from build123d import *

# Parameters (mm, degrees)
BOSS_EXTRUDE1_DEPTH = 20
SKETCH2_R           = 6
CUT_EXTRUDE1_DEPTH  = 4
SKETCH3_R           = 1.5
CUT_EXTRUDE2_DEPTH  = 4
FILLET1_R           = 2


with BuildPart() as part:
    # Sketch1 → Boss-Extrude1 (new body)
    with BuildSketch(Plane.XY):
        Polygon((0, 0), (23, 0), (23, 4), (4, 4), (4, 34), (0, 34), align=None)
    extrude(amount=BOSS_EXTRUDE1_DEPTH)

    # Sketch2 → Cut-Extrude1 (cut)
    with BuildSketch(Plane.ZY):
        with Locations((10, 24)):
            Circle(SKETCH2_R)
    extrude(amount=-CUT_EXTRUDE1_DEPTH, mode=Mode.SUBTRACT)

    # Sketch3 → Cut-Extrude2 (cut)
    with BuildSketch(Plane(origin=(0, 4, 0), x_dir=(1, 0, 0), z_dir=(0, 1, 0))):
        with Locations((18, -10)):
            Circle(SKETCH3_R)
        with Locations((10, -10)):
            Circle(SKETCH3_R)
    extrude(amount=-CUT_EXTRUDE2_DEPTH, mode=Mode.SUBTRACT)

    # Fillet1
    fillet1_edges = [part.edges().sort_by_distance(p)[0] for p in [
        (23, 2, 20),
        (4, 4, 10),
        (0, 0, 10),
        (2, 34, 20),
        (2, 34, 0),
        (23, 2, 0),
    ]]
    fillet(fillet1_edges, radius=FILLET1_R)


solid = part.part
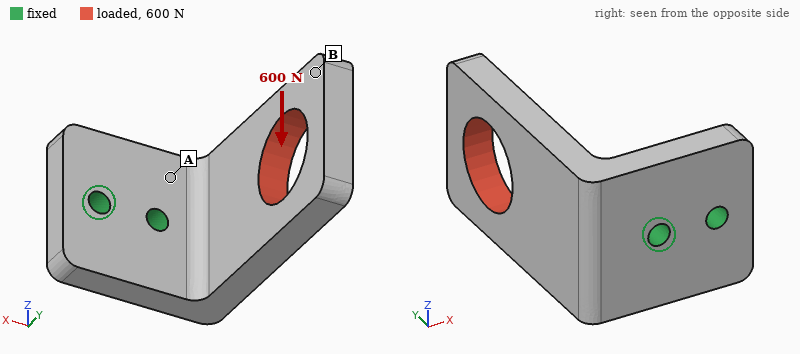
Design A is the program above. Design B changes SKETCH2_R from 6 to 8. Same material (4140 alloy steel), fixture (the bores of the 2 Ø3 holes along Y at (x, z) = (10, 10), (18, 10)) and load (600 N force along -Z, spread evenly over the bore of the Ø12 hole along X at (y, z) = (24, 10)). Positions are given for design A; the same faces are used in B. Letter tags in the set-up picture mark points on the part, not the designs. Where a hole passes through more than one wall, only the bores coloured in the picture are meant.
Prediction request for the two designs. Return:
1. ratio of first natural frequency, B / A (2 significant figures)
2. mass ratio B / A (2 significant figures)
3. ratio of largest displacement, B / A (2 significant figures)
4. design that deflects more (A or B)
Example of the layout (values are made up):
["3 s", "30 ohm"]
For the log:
["1.1", "0.91", "1.2", "B"]
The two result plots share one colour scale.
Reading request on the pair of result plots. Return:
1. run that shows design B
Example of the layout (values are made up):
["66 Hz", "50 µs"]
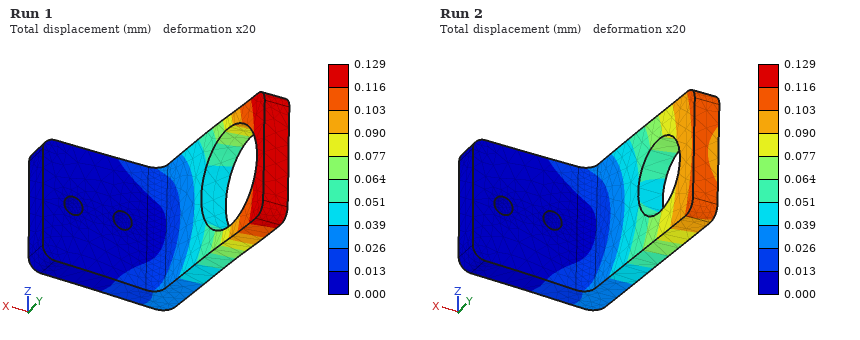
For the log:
["Run 1"]
